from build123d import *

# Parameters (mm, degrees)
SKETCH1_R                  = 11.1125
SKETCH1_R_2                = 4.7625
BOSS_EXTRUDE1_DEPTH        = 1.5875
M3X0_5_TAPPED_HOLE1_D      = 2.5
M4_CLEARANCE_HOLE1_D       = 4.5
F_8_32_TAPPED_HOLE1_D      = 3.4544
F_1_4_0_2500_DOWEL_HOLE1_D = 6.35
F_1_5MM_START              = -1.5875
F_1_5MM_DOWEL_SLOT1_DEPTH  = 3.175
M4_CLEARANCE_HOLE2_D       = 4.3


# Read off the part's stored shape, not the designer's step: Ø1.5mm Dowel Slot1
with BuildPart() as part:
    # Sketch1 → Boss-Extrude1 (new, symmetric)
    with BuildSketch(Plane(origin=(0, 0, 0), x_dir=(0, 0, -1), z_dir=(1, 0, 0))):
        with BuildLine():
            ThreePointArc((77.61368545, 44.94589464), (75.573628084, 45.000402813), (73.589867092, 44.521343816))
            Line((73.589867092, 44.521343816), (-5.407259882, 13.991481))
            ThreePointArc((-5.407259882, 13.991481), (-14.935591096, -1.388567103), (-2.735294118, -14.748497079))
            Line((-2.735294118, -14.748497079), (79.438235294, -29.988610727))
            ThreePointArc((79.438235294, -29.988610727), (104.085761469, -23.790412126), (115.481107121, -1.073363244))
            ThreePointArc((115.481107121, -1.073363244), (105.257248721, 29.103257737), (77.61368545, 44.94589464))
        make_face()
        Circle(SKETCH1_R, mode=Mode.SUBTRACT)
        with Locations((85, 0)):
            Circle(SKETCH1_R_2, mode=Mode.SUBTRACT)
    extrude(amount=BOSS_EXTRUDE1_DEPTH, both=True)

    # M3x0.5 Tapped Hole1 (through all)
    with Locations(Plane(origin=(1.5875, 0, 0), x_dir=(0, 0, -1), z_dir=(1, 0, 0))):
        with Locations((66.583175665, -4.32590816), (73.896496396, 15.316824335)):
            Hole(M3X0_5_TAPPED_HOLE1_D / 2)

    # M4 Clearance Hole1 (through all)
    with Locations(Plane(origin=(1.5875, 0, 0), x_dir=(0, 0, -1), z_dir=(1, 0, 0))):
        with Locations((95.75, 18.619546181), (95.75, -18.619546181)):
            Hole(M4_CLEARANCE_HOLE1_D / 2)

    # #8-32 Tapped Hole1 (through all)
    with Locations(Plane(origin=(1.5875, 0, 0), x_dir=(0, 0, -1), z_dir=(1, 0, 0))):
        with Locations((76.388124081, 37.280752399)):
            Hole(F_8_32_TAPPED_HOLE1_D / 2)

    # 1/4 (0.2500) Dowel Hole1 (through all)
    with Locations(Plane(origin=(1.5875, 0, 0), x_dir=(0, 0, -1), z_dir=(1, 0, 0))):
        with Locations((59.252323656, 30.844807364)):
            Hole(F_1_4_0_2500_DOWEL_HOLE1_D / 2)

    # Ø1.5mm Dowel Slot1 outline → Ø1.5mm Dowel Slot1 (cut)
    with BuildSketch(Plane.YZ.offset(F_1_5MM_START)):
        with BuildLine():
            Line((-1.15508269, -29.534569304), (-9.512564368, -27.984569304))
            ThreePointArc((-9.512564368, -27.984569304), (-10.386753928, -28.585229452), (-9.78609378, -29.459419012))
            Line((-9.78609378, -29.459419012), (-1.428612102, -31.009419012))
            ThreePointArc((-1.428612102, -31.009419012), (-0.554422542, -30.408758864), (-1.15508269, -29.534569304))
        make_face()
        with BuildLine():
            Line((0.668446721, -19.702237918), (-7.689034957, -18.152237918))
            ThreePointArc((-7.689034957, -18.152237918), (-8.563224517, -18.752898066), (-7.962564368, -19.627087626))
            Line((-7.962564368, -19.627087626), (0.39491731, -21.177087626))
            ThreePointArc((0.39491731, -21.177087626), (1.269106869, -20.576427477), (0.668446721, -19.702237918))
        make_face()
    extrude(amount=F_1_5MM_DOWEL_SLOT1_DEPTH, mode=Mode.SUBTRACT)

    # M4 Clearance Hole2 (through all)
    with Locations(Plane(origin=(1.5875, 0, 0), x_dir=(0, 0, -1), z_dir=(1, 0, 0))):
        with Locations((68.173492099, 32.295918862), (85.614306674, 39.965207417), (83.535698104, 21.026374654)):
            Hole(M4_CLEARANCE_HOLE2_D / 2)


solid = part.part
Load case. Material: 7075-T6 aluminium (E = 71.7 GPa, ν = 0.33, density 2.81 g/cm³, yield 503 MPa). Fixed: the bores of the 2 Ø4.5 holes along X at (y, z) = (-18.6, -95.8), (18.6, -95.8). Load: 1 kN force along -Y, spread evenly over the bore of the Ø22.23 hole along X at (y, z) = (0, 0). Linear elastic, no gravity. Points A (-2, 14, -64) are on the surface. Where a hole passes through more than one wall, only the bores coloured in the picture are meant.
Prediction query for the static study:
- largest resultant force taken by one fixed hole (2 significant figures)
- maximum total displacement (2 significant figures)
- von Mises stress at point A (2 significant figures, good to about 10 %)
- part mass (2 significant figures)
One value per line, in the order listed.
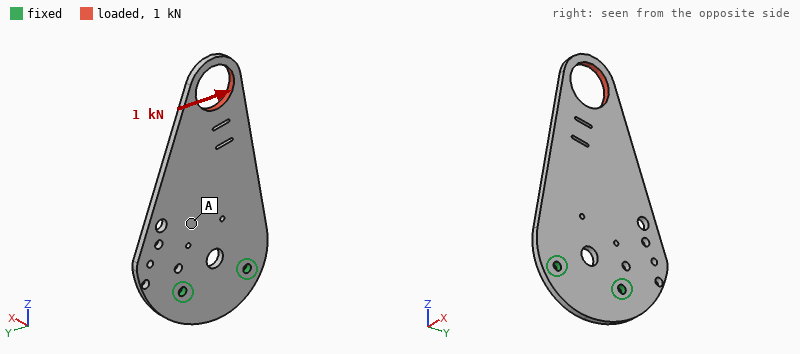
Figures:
2.5 kN
0.20 mm
15 MPa
55 g
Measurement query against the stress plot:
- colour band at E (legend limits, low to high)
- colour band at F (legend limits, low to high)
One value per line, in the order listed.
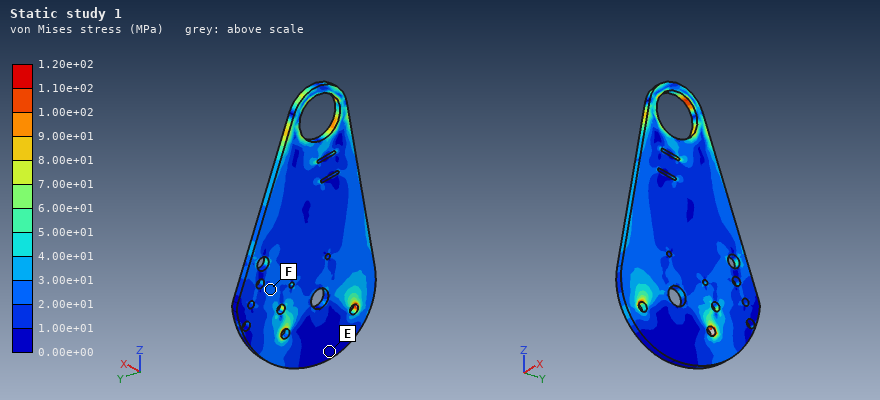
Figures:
0.00e+00 to 1.00e+01 MPa
2.00e+01 to 3.00e+01 MPa
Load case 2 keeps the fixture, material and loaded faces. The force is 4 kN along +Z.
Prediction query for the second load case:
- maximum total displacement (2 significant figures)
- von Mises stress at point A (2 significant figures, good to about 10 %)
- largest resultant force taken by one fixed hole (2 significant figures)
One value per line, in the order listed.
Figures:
0.10 mm
19 MPa
2.0 kN
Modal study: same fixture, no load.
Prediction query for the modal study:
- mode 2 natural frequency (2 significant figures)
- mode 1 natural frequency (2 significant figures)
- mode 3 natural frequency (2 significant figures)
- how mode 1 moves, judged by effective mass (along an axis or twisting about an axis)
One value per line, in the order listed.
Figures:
1300 Hz
330 Hz
1600 Hz
along X
